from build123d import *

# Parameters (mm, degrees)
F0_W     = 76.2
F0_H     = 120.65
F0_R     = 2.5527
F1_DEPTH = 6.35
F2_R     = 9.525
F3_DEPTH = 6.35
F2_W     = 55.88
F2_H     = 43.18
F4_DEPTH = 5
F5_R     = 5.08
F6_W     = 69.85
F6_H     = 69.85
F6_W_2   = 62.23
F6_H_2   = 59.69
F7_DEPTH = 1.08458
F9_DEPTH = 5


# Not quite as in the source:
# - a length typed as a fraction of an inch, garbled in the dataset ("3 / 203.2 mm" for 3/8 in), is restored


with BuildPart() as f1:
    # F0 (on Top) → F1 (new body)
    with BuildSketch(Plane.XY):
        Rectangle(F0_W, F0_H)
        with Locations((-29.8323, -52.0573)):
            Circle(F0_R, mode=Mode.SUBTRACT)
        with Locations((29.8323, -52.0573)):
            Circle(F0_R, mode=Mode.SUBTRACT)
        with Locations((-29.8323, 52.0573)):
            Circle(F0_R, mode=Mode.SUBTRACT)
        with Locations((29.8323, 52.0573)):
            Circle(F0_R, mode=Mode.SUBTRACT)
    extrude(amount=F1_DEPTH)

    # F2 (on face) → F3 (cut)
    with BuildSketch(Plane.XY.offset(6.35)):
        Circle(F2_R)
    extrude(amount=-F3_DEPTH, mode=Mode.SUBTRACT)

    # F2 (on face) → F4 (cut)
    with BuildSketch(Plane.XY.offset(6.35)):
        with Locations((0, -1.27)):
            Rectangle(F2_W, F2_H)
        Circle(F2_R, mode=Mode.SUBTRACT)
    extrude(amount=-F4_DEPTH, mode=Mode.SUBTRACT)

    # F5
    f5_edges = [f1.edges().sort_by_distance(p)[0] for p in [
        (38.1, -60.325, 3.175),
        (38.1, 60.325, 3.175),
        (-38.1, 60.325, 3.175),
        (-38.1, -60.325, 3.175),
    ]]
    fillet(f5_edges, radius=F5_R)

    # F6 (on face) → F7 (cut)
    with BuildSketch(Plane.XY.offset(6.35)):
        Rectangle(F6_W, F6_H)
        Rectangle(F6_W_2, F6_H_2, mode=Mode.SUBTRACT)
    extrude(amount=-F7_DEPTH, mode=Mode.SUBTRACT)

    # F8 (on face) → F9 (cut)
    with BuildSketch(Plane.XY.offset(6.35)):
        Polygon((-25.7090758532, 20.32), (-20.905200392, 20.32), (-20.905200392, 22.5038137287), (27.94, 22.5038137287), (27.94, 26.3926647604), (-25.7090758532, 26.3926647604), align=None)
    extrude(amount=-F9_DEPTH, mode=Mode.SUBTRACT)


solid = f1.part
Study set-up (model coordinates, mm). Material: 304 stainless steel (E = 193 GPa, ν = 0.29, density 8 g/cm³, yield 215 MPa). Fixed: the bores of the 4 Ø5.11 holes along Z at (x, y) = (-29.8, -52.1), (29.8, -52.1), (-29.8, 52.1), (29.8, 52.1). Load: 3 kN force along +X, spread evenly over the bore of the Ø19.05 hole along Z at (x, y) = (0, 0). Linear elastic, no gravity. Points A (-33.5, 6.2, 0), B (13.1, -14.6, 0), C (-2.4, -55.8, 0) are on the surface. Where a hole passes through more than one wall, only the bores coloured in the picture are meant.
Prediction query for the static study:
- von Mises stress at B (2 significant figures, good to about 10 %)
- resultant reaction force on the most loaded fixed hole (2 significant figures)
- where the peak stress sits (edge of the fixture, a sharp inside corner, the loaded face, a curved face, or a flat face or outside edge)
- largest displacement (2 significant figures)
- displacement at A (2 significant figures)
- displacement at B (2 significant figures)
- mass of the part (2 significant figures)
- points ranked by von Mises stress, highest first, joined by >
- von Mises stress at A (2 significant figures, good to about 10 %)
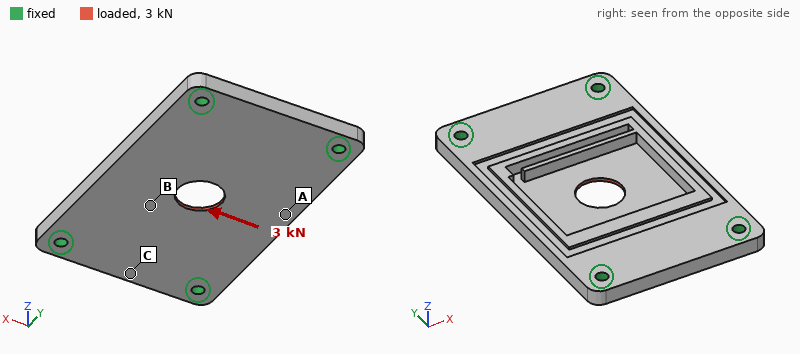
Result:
27 MPa
1.0 kN
the loaded face
7.7 µm
4.9 µm
4.2 µm
340 g
B > A > C
12 MPa
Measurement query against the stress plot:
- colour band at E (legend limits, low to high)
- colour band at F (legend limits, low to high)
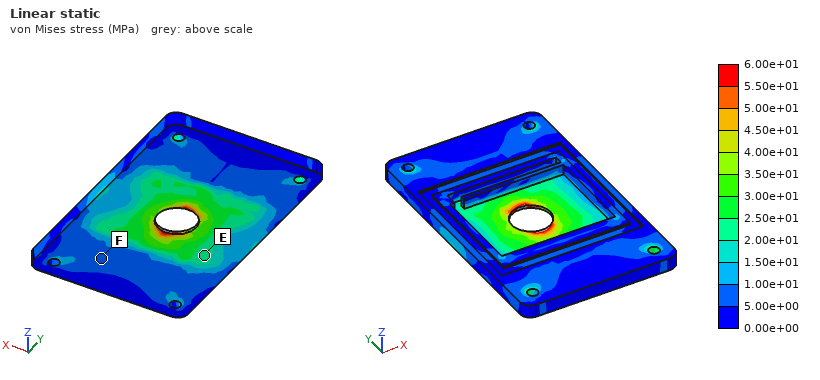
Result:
2.00e+01 to 2.50e+01 MPa
5.00e+00 to 1.00e+01 MPa
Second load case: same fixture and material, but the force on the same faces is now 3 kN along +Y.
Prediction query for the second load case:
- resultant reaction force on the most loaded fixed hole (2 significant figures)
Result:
790 N
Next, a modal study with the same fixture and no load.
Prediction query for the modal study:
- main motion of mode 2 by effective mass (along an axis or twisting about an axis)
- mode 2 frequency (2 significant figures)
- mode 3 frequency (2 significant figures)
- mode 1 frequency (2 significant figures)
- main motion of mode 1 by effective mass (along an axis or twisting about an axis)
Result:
twisting about Y
3700 Hz
4900 Hz
2900 Hz
along Z
